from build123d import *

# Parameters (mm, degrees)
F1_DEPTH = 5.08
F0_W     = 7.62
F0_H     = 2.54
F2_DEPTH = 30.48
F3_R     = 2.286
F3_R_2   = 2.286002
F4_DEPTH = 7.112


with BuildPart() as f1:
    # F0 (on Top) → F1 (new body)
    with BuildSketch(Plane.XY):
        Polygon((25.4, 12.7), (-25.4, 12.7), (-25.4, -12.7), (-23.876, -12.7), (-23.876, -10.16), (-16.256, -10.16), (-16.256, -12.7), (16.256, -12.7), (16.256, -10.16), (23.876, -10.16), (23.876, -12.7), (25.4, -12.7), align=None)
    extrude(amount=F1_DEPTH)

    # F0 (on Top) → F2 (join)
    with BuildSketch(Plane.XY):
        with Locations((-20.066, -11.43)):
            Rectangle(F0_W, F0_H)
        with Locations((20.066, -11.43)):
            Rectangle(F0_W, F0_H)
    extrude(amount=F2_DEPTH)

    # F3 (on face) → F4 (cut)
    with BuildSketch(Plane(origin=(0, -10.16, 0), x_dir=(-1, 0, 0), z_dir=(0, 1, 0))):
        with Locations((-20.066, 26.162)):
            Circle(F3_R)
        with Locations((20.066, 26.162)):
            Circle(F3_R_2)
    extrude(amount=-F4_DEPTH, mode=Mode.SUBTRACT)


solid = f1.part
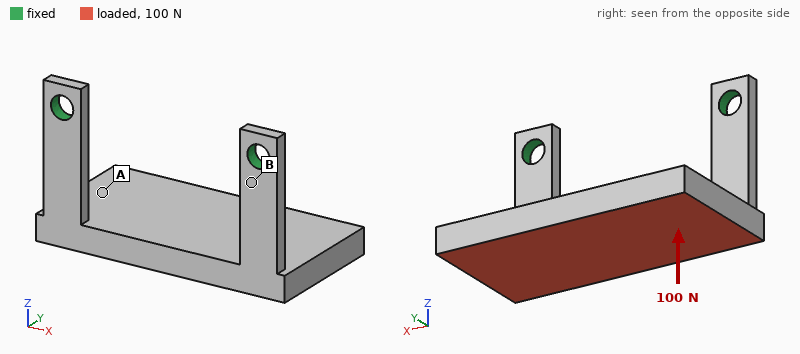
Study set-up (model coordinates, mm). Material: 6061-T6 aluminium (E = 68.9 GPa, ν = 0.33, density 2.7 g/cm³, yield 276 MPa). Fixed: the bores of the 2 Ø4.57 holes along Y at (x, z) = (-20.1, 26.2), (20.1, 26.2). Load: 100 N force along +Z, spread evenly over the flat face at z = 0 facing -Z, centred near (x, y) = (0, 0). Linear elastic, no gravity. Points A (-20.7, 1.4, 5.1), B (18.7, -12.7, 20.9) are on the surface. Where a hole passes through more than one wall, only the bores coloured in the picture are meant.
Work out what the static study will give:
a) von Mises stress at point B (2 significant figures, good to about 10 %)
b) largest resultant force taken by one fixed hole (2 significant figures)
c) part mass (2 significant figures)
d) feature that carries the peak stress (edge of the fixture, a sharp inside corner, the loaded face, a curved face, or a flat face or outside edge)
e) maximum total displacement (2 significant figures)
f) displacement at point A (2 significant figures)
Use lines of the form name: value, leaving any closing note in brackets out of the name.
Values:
von Mises stress at point B: 66 MPa
largest resultant force taken by one fixed hole: 51 N
part mass: 20 g
feature that carries the peak stress: a flat face or outside edge
maximum total displacement: 0.46 mm
displacement at point A: 0.25 mm
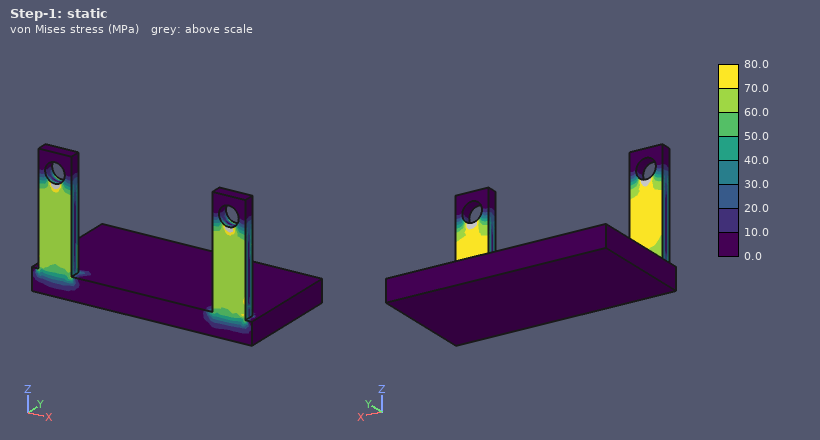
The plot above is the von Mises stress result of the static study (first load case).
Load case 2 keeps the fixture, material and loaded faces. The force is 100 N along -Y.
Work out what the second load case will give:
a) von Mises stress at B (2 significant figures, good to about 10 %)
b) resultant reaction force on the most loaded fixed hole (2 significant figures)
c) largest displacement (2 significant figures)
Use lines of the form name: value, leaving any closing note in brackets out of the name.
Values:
von Mises stress at B: 120 MPa
resultant reaction force on the most loaded fixed hole: 50 N
largest displacement: 0.59 mm
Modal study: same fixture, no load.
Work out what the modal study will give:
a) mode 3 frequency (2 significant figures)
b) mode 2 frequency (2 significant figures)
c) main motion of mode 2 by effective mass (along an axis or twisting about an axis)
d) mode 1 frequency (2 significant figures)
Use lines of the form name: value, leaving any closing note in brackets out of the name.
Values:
mode 3 frequency: 2200 Hz
mode 2 frequency: 1600 Hz
main motion of mode 2 by effective mass: along X
mode 1 frequency: 550 Hz
